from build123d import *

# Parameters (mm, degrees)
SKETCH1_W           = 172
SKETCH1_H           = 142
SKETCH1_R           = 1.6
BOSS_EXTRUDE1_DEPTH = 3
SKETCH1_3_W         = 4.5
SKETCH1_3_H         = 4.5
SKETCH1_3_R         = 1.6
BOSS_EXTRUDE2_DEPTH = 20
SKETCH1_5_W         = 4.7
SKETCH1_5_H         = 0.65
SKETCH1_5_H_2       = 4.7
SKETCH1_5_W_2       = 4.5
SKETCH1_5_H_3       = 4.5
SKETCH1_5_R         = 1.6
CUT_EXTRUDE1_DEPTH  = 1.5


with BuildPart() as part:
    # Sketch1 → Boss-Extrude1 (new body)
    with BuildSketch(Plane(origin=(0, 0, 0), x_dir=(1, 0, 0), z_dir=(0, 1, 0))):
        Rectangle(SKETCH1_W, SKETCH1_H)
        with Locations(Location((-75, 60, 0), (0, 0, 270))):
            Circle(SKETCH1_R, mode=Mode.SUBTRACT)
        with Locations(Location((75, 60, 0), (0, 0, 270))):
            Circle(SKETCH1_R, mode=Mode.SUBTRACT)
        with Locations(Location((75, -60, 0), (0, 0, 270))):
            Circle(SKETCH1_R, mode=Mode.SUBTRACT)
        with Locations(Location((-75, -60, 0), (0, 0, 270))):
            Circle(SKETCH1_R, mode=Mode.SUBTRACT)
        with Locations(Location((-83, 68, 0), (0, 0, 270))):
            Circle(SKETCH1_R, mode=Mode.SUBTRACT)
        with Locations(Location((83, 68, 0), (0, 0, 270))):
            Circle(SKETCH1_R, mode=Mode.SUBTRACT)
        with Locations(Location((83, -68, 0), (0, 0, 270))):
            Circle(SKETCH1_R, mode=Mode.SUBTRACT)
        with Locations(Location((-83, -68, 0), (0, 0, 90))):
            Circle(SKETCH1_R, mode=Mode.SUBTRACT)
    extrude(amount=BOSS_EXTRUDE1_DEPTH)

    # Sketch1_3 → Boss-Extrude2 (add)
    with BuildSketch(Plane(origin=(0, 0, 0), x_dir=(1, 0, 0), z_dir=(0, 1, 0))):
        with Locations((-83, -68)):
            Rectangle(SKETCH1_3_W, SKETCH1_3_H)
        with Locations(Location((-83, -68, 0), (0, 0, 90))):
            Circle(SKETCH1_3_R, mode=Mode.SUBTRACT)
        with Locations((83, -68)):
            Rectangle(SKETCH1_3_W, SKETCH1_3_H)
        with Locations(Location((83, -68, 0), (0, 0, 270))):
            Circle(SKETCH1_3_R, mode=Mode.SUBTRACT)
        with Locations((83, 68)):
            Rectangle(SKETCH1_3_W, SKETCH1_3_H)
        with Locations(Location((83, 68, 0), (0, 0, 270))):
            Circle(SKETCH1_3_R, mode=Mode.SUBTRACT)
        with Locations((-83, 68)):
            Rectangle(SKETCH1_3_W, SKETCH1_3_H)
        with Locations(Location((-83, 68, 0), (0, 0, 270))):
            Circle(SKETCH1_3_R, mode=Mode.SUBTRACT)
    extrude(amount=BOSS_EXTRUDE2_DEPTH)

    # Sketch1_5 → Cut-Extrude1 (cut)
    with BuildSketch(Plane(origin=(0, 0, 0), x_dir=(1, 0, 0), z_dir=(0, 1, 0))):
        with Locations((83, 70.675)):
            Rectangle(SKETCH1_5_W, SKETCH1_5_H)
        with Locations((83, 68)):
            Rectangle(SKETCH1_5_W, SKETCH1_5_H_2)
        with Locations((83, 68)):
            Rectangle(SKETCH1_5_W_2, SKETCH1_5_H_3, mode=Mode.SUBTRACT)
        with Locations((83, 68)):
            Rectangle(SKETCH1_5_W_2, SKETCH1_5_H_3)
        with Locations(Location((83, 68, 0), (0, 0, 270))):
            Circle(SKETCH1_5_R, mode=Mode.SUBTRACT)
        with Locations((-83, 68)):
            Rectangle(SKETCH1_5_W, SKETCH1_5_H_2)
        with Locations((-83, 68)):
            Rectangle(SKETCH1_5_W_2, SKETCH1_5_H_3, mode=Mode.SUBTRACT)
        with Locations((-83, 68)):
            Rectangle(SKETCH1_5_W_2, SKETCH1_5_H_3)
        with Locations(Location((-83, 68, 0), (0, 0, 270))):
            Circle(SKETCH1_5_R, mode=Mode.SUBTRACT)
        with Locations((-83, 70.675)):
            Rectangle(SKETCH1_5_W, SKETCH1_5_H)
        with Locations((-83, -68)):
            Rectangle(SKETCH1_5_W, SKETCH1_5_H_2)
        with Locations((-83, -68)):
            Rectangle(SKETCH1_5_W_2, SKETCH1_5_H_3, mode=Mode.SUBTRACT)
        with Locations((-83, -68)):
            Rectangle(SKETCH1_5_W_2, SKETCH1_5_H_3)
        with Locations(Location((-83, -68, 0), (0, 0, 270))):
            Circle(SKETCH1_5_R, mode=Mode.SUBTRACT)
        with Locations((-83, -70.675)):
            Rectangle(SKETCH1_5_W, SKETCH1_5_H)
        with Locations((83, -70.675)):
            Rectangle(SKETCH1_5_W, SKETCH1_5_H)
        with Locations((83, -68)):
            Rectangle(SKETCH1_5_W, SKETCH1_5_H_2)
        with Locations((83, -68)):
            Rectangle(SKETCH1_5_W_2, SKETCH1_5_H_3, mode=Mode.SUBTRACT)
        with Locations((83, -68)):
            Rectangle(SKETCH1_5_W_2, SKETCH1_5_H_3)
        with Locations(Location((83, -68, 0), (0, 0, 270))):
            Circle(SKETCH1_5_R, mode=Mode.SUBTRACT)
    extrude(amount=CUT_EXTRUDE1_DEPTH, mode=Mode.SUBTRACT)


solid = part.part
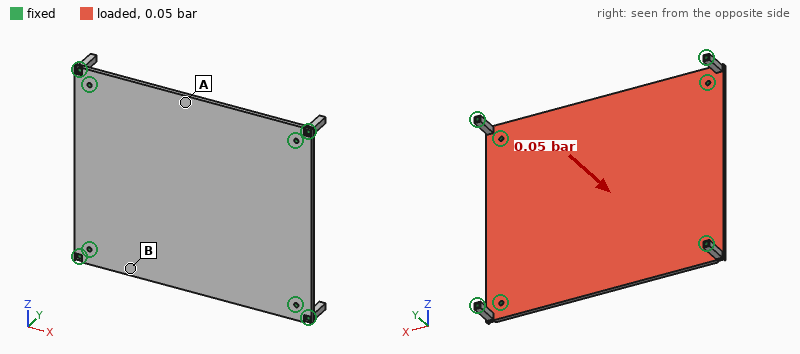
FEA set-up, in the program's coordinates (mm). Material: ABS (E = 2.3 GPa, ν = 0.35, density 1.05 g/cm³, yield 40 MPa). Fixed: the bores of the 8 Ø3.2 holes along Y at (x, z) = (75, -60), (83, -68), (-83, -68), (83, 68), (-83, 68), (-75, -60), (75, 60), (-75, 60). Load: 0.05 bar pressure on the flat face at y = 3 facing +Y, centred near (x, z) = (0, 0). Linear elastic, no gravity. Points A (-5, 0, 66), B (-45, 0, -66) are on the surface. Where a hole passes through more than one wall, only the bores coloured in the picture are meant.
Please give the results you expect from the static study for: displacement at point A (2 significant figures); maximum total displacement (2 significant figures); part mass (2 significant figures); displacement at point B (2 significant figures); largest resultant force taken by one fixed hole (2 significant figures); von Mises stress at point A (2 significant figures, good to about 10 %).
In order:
1.9 mm
2.6 mm
77 g
0.78 mm
52 N
4.5 MPa
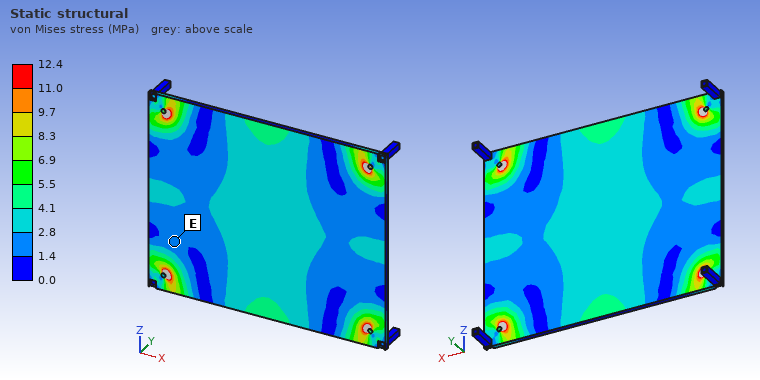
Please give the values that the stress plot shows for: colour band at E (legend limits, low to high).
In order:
1.4 to 2.8 MPa
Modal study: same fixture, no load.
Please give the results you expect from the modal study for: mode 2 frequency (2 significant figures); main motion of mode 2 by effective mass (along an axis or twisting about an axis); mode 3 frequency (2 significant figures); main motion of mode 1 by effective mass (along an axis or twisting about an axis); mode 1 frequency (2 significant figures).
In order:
240 Hz
twisting about X
310 Hz
along Y
150 Hz
